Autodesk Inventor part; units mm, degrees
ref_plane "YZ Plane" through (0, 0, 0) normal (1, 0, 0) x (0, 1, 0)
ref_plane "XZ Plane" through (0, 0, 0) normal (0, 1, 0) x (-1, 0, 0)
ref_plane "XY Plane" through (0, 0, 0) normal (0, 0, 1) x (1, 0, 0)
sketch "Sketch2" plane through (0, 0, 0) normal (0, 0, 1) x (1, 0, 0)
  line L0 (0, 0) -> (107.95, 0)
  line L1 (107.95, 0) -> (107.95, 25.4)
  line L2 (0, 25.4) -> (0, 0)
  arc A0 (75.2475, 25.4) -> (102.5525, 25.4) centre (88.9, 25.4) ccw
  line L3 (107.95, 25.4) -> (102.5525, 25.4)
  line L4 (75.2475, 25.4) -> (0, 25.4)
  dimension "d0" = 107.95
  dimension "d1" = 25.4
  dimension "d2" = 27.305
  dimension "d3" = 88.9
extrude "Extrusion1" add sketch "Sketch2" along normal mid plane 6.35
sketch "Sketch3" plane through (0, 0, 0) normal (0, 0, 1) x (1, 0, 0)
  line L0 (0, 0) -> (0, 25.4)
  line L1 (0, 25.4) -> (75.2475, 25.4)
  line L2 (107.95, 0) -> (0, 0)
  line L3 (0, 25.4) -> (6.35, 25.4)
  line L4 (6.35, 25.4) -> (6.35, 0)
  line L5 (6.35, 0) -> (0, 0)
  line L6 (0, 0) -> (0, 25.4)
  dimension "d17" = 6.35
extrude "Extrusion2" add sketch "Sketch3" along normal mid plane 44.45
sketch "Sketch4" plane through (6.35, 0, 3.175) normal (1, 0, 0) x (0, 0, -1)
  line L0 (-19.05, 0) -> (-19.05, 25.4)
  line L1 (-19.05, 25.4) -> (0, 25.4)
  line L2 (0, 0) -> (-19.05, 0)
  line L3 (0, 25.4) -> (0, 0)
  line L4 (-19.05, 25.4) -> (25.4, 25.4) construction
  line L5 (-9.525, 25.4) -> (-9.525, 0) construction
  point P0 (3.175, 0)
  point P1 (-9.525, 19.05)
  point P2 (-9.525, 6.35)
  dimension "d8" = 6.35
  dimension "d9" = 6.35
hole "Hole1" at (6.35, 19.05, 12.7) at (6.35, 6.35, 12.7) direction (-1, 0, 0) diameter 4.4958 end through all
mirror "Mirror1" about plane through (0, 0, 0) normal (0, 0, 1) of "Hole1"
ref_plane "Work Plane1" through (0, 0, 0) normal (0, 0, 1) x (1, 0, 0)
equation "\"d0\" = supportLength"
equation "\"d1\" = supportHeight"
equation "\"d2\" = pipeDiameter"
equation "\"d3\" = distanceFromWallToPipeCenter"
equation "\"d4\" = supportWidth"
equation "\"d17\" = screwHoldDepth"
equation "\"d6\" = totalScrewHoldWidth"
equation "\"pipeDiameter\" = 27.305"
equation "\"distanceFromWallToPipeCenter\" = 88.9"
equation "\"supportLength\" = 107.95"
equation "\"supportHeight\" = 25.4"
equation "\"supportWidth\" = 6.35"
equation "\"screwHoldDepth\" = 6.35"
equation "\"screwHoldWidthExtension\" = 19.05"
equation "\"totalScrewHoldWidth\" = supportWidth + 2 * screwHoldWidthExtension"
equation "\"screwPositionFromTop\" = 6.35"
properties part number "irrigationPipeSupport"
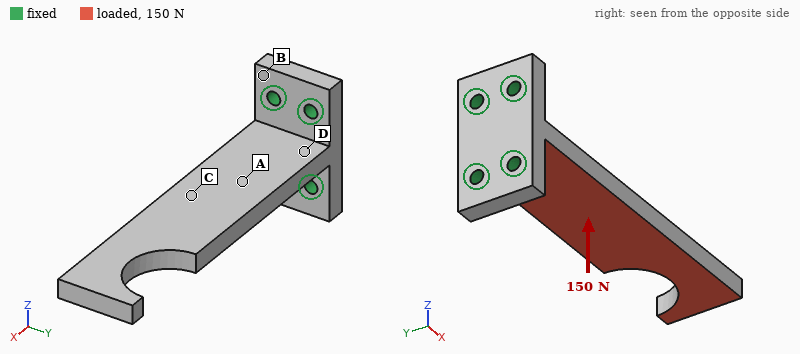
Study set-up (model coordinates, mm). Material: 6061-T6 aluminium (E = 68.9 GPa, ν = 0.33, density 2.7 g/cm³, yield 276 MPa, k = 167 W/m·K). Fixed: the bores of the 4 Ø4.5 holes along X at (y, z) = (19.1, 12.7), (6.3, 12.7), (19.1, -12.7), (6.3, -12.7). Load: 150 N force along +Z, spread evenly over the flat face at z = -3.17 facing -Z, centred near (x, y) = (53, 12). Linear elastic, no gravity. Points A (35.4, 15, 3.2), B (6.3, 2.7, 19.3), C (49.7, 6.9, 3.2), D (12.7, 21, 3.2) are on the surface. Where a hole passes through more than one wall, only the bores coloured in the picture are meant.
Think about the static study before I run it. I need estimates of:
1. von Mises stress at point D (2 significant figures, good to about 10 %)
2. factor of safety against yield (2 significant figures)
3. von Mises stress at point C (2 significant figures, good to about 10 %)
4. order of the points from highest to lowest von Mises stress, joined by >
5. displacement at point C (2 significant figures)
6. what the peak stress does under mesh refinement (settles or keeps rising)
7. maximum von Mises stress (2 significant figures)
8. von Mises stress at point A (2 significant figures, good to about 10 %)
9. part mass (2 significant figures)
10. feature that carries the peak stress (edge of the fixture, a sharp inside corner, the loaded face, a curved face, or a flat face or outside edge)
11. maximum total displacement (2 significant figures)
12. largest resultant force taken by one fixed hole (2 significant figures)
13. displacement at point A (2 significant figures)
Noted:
34 MPa
7.5
12 MPa
D > A > C > B
0.15 mm
settles
37 MPa
20 MPa
57 g
the loaded face
0.52 mm
220 N
0.081 mm
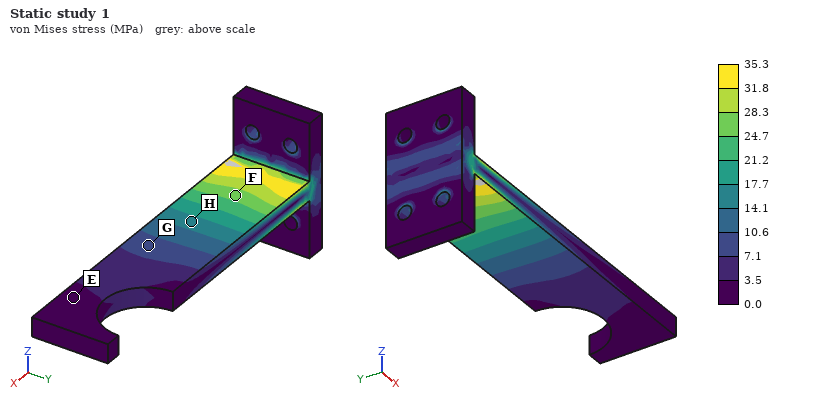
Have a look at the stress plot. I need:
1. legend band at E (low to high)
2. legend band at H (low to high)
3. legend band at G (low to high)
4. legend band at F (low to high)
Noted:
0.0 to 3.5 MPa
14.1 to 17.7 MPa
7.1 to 10.6 MPa
24.7 to 28.3 MPa
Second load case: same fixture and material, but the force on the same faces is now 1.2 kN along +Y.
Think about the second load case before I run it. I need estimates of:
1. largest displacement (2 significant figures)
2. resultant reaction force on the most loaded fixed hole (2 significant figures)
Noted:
0.54 mm
1.8 kN
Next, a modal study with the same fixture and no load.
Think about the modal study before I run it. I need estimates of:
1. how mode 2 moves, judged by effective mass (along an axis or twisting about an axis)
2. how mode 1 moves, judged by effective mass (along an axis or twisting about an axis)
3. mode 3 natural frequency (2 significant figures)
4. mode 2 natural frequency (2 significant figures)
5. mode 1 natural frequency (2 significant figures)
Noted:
along Y
along Z
2800 Hz
1500 Hz
550 Hz
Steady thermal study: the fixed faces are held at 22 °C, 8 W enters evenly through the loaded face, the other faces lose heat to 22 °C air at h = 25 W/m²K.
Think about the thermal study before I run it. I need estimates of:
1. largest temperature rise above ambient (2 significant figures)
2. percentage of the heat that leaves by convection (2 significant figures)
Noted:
14 K
12 %
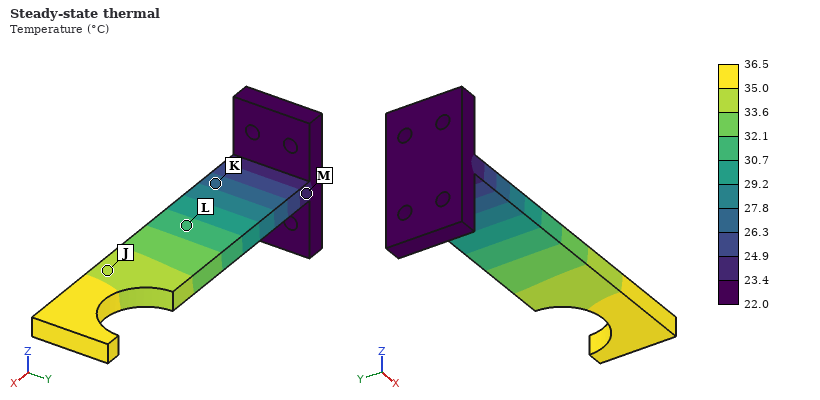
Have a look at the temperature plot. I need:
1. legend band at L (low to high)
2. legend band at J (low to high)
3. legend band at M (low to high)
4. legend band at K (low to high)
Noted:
30.7 to 32.1 °C
33.6 to 35.0 °C
23.4 to 24.9 °C
26.3 to 27.8 °C
